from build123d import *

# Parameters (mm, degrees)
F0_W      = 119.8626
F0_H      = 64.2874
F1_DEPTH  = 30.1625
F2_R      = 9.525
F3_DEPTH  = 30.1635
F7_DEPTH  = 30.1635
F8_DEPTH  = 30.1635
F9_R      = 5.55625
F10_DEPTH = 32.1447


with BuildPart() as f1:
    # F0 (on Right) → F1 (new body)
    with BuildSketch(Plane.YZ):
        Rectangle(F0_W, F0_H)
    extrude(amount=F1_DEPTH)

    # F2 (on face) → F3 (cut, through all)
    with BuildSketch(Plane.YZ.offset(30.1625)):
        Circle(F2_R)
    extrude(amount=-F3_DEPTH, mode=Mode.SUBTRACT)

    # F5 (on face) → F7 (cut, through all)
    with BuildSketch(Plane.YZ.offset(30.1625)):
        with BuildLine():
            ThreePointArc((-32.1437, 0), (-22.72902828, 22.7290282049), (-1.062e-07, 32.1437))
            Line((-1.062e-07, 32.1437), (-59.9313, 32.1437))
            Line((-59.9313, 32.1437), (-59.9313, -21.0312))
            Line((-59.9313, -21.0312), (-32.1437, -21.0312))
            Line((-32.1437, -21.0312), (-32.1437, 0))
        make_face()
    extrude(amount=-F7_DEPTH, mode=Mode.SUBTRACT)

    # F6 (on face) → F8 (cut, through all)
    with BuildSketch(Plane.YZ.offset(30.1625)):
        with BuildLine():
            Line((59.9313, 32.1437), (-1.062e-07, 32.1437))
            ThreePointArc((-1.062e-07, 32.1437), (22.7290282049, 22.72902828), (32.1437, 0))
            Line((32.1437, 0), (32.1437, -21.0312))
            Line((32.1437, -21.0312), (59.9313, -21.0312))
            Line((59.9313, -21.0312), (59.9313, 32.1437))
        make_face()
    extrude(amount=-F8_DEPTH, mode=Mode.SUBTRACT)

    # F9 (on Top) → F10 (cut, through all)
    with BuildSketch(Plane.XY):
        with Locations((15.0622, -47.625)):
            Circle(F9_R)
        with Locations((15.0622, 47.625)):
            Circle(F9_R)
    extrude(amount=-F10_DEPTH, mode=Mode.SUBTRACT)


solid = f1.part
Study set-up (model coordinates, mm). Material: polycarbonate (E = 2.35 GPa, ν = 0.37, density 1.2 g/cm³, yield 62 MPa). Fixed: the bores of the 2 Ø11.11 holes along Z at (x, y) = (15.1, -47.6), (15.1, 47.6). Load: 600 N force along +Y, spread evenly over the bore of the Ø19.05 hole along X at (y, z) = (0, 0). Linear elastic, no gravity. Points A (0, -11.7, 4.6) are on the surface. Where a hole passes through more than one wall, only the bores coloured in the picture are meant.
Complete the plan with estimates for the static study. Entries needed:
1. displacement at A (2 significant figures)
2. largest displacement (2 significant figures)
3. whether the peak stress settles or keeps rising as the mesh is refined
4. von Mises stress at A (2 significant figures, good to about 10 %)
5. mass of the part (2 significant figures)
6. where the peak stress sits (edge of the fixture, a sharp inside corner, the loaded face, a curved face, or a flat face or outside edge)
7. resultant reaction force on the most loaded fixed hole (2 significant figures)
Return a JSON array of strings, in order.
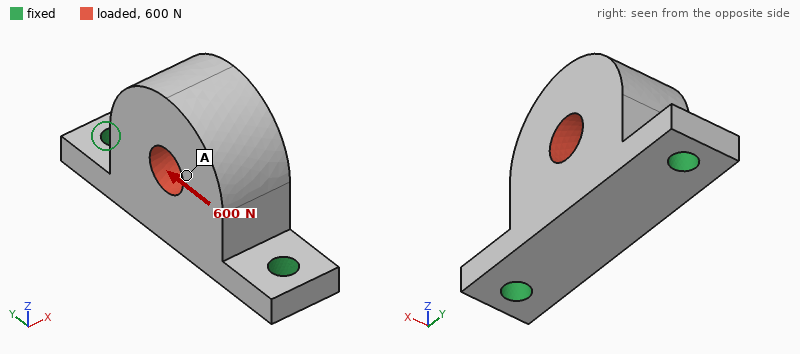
["41 µm", "59 µm", "keeps rising", "0.58 MPa", "140 g", "edge of the fixture", "370 N"]
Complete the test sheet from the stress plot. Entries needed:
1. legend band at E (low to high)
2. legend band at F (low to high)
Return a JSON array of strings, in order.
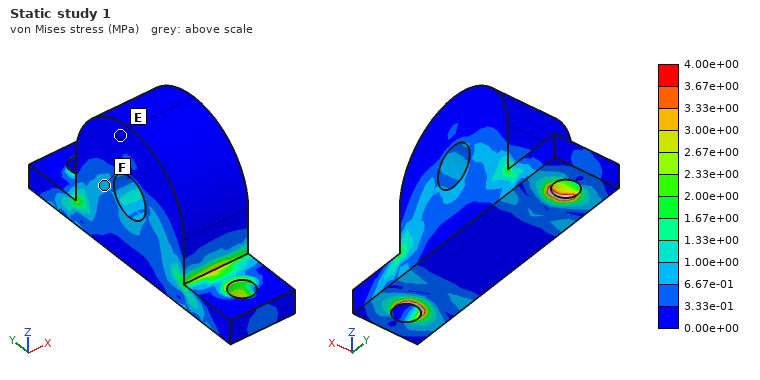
["0.00e+00 to 3.33e-01 MPa", "6.67e-01 to 1.00e+00 MPa"]
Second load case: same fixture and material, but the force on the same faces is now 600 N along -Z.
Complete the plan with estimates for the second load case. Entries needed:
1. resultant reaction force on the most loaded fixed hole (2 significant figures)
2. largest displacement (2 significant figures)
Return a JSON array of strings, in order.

["340 N", "53 µm"]
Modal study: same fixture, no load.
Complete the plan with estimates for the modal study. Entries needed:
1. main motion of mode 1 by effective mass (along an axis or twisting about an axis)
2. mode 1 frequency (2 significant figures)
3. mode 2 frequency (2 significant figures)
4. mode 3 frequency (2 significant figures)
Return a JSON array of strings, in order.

["along X", "530 Hz", "1600 Hz", "1700 Hz"]
